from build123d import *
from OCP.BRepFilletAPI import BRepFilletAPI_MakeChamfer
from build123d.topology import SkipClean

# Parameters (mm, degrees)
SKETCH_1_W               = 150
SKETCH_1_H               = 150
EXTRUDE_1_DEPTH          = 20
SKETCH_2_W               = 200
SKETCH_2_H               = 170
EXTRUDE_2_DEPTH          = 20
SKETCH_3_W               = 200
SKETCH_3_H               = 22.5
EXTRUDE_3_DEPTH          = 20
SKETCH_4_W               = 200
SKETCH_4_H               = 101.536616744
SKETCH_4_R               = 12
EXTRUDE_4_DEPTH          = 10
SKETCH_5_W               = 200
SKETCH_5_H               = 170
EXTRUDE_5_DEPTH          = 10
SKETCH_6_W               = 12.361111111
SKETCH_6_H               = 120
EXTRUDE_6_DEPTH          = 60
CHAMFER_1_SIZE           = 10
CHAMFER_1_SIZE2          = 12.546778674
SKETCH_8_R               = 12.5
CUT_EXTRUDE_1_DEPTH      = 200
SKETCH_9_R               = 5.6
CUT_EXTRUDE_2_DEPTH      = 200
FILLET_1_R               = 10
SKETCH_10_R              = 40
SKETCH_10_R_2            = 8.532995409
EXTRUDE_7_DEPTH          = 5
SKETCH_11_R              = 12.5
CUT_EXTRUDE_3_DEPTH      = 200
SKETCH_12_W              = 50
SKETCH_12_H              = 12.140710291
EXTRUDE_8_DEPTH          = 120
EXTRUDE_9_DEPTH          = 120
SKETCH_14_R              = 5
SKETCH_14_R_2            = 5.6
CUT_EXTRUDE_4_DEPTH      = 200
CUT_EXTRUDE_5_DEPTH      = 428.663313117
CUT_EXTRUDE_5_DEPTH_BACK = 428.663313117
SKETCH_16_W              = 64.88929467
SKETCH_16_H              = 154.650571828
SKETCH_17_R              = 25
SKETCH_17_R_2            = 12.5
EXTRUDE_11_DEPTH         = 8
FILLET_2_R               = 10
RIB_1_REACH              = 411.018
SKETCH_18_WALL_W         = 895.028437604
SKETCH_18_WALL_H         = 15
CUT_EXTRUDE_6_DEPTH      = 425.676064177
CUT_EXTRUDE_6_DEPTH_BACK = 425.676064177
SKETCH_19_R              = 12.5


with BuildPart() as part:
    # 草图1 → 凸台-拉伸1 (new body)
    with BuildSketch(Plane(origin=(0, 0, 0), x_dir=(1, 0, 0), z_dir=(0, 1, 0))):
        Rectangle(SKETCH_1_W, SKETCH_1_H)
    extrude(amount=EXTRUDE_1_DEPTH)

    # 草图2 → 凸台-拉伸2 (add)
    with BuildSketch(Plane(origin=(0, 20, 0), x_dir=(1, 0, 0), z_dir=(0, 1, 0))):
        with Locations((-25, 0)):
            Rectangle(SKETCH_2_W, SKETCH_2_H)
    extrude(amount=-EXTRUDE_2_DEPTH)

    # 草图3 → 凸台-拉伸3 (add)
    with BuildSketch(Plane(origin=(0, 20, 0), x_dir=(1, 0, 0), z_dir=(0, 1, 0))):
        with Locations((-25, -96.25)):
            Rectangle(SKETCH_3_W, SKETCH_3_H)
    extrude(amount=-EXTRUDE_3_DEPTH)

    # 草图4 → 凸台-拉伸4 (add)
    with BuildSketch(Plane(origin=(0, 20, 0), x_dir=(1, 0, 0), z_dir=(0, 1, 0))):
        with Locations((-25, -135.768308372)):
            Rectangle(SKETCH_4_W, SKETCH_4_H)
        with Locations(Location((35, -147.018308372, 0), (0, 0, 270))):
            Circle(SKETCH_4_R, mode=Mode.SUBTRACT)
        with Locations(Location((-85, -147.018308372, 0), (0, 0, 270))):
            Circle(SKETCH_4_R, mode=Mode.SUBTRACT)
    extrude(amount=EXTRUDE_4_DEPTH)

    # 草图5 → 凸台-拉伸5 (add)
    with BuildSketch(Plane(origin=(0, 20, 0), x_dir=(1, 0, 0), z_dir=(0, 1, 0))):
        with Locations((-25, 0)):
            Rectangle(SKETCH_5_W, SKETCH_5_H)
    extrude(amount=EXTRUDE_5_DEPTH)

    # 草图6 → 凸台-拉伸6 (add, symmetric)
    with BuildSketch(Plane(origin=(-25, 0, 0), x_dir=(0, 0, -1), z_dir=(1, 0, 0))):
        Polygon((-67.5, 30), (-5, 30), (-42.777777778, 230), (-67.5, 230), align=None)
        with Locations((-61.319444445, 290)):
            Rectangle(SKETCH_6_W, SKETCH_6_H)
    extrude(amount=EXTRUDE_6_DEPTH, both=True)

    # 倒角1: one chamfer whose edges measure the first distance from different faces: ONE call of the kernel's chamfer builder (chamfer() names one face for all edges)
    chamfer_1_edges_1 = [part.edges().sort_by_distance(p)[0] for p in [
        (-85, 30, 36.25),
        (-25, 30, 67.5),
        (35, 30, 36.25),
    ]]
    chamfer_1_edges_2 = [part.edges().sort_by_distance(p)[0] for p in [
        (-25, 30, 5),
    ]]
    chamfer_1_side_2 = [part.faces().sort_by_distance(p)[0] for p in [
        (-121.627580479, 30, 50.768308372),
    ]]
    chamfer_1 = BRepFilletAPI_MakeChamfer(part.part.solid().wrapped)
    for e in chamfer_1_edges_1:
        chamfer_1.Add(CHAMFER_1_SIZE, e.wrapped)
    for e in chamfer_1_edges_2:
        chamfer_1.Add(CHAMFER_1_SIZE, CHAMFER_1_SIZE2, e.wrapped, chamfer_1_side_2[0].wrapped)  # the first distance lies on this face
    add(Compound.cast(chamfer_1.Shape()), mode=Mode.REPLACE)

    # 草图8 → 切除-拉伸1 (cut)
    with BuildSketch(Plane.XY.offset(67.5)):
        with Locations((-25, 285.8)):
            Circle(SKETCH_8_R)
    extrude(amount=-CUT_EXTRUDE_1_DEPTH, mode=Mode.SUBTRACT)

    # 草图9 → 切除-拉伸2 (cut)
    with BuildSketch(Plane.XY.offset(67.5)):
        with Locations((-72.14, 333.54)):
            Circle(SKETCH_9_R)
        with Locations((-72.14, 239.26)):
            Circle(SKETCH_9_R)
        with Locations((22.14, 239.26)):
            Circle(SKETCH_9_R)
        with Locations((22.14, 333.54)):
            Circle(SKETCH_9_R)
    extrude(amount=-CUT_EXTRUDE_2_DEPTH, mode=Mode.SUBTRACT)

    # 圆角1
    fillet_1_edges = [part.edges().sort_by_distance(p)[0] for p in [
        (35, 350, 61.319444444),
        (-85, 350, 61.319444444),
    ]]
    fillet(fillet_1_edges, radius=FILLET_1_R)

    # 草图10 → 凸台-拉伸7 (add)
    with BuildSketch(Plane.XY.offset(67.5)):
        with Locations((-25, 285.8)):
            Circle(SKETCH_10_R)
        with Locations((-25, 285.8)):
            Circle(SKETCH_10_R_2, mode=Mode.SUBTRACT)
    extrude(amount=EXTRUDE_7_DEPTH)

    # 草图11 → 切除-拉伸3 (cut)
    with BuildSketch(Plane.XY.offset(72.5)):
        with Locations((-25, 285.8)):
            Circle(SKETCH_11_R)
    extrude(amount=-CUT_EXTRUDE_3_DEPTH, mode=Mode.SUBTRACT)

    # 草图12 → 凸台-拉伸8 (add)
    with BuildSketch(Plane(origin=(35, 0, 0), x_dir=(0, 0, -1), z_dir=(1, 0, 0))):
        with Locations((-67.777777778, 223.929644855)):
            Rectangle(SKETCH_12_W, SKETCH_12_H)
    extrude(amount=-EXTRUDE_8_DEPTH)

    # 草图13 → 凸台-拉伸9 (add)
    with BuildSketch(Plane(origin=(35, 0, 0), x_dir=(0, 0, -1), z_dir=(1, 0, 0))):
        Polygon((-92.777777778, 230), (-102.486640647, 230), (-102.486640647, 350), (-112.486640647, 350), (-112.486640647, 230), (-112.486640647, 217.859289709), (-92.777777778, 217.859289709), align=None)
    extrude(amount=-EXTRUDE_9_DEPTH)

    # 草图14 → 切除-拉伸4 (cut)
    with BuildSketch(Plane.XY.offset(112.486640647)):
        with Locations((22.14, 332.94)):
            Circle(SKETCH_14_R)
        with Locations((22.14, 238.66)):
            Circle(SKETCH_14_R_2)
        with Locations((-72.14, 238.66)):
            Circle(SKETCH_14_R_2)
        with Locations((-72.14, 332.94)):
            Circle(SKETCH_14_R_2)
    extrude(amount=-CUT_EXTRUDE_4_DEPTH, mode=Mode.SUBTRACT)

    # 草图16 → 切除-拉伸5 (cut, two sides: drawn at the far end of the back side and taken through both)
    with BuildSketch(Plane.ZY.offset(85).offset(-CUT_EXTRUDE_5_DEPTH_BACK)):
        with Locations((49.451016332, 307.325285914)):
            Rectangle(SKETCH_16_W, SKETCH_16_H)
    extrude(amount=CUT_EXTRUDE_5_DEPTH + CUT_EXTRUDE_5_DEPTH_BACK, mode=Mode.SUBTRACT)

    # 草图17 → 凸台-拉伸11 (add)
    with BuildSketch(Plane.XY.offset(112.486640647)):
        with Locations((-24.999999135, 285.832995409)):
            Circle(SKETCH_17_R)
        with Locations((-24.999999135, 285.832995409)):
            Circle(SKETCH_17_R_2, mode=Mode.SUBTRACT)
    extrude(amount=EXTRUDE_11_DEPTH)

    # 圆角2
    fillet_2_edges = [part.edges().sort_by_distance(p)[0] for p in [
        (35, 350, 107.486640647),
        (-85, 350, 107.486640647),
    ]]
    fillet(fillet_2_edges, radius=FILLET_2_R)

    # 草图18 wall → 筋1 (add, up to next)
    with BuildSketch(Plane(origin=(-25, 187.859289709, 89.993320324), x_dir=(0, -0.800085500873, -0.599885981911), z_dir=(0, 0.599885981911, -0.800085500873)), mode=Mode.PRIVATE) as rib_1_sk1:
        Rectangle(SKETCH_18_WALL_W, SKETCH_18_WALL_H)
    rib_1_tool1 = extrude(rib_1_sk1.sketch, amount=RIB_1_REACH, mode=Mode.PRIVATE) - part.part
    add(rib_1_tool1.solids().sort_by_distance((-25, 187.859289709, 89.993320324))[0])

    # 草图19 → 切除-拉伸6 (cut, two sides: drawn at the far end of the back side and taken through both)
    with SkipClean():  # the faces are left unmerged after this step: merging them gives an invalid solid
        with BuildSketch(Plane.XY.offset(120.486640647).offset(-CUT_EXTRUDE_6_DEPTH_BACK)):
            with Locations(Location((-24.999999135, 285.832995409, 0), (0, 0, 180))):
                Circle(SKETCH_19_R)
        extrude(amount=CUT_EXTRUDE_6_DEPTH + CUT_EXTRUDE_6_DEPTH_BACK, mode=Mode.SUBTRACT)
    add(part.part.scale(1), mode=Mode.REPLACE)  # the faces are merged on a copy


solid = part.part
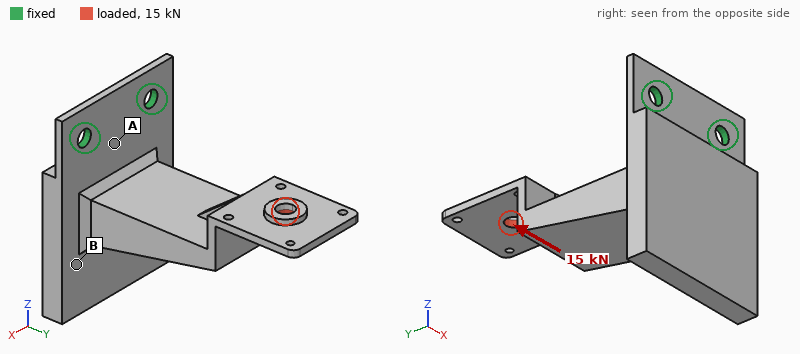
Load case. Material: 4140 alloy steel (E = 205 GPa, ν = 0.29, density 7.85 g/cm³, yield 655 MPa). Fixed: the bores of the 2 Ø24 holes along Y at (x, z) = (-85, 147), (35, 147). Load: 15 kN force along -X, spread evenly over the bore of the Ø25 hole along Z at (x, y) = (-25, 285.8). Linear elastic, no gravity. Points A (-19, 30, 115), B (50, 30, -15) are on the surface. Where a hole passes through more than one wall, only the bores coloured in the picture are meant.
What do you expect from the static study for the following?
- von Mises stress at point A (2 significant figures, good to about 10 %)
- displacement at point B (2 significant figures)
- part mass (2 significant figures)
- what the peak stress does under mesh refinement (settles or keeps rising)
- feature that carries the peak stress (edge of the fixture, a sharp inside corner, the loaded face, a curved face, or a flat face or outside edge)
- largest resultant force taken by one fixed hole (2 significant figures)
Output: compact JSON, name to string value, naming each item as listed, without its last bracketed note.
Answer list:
{"von Mises stress at point A": "86 MPa", "displacement at point B": "0.27 mm", "part mass": "20 kg", "what the peak stress does under mesh refinement": "keeps rising", "feature that carries the peak stress": "edge of the fixture", "largest resultant force taken by one fixed hole": "31 kN"}
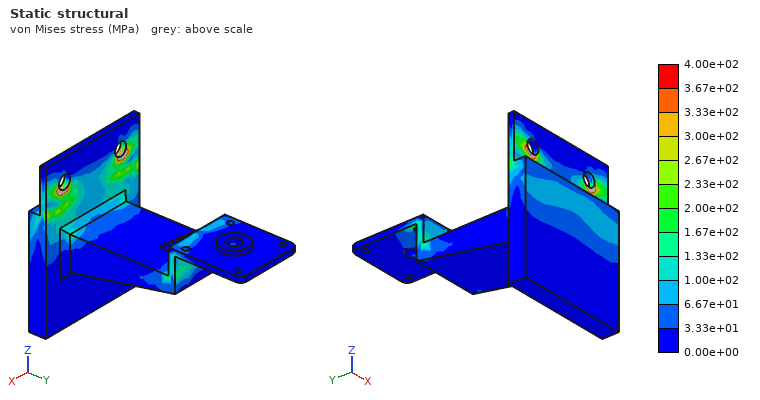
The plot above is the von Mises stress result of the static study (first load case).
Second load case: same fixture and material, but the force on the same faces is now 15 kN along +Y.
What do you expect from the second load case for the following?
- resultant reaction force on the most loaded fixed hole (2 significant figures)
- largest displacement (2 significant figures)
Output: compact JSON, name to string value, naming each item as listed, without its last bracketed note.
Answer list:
{"resultant reaction force on the most loaded fixed hole": "7.5 kN", "largest displacement": "0.53 mm"}
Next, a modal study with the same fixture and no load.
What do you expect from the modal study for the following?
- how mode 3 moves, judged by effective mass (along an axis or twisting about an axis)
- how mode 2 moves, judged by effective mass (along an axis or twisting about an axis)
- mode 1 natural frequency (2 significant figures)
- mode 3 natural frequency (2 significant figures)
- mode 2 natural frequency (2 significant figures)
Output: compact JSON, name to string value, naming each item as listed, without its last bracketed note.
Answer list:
{"how mode 3 moves, judged by effective mass": "along Y", "how mode 2 moves, judged by effective mass": "along X", "mode 1 natural frequency": "75 Hz", "mode 3 natural frequency": "460 Hz", "mode 2 natural frequency": "330 Hz"}
